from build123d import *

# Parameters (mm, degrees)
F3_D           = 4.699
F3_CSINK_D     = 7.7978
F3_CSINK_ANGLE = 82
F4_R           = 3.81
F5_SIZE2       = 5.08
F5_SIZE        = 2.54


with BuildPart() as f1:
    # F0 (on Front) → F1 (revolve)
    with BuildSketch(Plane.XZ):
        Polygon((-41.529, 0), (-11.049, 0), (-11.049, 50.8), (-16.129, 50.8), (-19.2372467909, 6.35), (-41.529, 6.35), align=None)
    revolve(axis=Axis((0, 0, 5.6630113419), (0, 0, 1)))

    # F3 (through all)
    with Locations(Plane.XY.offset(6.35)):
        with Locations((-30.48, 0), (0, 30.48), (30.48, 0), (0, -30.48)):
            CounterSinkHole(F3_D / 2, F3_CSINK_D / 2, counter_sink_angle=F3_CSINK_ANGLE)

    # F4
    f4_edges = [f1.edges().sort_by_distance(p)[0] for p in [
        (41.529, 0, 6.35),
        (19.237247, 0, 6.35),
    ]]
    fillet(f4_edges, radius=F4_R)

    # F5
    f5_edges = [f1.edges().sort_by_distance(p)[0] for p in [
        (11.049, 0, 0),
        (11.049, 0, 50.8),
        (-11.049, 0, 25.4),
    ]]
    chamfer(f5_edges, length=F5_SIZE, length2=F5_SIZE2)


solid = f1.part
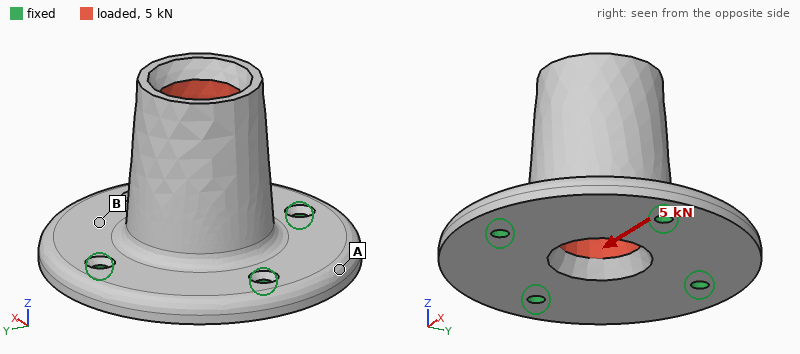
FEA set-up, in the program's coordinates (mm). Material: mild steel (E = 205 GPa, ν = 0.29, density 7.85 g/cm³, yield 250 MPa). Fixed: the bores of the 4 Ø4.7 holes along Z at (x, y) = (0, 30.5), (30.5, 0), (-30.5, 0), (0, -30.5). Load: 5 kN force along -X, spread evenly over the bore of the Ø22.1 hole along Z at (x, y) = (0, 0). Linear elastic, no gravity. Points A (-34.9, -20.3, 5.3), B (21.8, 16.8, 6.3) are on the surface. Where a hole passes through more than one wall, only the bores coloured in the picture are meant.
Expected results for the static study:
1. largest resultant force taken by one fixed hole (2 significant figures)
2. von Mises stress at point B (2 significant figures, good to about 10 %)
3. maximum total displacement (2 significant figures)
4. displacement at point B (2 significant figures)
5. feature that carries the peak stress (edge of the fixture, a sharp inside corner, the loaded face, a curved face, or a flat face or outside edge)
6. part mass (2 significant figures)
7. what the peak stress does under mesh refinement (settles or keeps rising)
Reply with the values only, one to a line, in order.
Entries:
2.7 kN
18 MPa
20 µm
4.2 µm
edge of the fixture
450 g
keeps rising
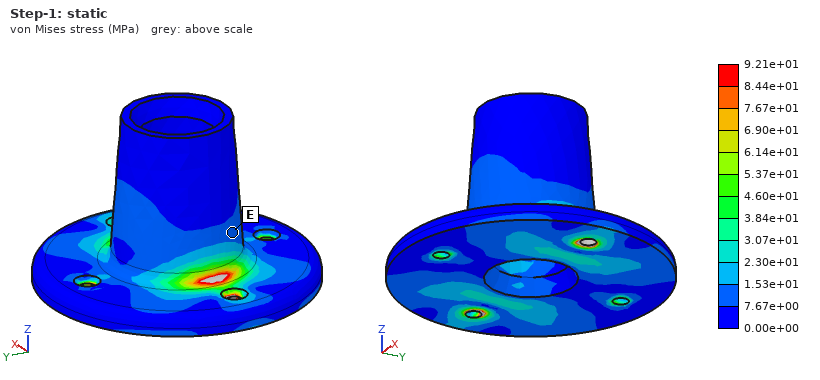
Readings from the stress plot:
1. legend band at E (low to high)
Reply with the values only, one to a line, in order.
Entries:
7.67e+00 to 1.53e+01 MPa
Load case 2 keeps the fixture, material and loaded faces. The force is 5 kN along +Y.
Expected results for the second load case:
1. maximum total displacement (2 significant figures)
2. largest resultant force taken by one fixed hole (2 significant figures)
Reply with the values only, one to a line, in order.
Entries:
20 µm
2.7 kN
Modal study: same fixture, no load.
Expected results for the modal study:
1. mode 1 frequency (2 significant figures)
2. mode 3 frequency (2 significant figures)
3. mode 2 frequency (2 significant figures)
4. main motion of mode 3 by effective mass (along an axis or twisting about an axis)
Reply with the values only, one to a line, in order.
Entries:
6200 Hz
8900 Hz
6200 Hz
along Z
